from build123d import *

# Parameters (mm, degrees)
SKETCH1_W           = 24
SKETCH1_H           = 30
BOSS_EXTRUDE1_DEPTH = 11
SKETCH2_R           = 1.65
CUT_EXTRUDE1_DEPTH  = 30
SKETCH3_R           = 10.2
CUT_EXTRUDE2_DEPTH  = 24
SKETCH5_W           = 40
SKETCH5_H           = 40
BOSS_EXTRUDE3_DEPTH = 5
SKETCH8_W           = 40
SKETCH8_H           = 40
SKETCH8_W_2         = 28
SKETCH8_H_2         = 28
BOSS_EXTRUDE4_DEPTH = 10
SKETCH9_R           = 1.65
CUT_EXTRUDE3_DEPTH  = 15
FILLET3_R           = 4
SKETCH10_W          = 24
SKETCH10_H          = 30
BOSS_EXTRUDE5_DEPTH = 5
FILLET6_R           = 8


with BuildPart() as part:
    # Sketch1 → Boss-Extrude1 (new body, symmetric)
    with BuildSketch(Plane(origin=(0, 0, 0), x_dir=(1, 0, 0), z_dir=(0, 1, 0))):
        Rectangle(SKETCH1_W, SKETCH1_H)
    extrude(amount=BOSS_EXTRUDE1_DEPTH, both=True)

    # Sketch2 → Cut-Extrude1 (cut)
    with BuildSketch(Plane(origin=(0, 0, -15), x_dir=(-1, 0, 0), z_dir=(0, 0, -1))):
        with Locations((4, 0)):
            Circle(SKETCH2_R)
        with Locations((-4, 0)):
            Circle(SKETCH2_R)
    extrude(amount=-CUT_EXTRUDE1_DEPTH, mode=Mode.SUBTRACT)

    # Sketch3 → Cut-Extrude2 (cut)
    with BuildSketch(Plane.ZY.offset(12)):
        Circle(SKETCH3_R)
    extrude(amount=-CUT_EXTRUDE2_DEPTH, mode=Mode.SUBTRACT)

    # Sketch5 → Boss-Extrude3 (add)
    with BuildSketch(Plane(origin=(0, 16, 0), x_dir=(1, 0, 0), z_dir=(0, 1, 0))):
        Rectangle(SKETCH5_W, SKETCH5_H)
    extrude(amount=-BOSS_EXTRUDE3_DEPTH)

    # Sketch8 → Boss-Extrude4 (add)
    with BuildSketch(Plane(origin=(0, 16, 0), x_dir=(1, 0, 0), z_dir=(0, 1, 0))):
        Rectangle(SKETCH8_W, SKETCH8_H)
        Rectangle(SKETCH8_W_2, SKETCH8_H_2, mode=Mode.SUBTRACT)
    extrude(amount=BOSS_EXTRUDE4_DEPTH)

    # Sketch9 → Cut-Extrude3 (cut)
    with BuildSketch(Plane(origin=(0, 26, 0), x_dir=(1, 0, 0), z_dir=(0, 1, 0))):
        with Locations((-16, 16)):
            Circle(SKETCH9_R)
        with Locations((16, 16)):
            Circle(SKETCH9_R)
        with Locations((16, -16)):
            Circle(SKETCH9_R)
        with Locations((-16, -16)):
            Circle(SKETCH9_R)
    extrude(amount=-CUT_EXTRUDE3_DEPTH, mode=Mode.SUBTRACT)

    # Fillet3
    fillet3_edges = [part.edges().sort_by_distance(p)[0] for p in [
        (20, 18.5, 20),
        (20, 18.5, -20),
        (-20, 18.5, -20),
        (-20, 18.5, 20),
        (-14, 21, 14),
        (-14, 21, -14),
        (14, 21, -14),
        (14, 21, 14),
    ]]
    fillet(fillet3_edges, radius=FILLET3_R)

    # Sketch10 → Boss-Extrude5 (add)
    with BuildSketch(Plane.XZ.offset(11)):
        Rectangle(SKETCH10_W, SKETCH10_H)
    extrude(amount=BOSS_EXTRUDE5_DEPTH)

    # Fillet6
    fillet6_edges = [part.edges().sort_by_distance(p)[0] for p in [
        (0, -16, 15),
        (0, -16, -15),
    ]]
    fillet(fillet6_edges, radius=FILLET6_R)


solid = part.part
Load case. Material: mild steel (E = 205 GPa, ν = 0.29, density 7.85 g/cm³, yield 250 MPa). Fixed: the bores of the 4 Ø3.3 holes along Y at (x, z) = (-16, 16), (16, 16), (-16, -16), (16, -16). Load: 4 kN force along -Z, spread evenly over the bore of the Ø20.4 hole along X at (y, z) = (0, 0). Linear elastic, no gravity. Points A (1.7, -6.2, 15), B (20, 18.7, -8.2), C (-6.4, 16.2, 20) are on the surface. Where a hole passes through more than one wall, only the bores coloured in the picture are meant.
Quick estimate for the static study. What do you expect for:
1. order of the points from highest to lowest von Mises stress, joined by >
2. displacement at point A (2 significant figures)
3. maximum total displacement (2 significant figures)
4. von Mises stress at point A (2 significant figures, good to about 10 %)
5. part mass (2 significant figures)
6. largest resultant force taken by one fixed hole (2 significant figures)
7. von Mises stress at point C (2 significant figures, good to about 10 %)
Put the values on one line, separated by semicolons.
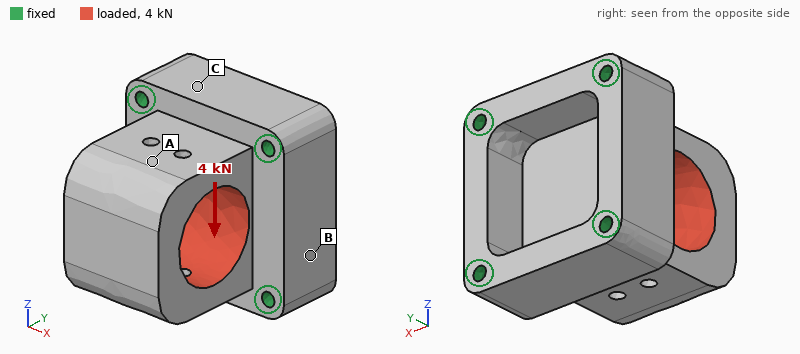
A > C > B; 11 µm; 13 µm; 21 MPa; 210 g; 1.5 kN; 12 MPa
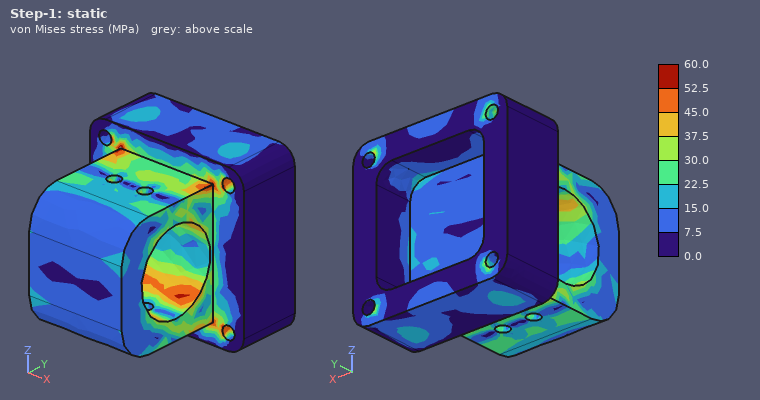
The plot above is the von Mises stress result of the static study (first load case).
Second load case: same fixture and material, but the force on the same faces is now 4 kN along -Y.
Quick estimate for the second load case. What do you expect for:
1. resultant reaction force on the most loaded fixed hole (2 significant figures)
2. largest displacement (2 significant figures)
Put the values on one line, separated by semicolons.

1.1 kN; 3.1 µm
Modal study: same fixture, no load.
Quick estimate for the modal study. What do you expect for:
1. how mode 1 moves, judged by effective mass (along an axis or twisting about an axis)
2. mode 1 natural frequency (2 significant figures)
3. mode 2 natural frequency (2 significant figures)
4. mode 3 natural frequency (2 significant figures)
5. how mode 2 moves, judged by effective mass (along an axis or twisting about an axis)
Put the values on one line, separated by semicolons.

along Z; 9200 Hz; 11 kHz; 17 kHz; along X
